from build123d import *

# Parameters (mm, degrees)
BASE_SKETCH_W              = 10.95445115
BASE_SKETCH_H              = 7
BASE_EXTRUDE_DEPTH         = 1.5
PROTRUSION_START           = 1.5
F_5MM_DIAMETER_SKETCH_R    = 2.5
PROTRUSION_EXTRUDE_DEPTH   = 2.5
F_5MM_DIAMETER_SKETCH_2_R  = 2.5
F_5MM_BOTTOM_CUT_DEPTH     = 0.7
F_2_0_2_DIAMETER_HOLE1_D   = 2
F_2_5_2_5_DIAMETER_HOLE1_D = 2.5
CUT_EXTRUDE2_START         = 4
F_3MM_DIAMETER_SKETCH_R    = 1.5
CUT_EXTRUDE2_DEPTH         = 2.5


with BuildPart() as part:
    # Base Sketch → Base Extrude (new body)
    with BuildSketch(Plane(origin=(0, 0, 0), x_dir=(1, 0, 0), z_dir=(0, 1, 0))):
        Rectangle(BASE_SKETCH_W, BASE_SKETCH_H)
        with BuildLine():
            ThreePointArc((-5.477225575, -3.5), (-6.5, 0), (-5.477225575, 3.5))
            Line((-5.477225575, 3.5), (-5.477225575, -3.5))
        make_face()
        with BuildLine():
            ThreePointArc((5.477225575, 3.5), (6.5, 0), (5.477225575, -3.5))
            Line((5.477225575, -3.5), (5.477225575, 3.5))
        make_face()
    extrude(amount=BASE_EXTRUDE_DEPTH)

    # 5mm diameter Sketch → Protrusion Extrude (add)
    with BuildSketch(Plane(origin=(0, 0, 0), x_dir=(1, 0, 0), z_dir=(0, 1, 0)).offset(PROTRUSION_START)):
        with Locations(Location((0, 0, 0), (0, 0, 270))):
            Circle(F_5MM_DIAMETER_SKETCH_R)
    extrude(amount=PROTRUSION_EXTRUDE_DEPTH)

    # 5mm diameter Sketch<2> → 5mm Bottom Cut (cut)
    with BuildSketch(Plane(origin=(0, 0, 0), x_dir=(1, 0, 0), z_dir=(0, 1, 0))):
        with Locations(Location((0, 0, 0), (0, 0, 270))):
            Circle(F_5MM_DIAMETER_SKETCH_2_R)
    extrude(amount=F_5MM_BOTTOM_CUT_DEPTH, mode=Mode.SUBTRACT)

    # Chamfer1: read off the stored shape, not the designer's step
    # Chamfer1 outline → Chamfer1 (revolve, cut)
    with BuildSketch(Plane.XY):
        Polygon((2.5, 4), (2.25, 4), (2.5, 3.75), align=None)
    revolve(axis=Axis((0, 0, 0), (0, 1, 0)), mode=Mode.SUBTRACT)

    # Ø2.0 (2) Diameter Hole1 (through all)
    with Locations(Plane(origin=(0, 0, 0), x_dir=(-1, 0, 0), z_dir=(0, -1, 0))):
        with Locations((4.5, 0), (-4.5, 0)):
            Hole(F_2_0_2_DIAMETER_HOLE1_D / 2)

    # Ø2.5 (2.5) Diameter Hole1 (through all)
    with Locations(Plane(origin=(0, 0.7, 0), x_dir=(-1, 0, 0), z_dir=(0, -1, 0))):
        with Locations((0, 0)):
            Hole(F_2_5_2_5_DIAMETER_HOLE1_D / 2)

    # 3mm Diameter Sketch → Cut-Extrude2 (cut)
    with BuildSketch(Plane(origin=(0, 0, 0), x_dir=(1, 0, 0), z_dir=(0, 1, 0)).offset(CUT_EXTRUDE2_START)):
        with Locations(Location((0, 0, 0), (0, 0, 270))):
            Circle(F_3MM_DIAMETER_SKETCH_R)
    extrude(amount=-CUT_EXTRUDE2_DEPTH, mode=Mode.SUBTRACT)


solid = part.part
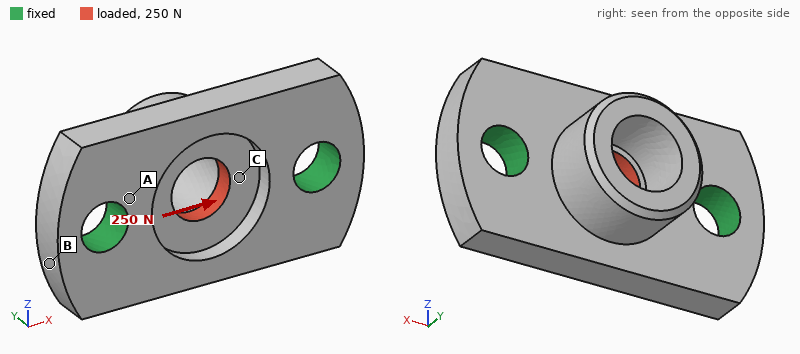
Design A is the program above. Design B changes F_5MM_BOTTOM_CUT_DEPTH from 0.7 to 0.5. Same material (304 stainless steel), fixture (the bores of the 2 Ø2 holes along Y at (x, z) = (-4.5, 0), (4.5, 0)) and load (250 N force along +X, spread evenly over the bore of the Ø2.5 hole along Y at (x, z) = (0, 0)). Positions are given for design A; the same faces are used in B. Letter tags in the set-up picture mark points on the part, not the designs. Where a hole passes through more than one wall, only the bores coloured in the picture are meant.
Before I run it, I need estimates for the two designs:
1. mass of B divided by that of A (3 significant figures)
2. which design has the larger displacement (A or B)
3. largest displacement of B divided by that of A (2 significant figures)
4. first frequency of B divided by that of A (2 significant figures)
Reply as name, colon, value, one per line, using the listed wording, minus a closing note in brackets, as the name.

mass of B divided by that of A: 1.02
which design has the larger displacement: A
largest displacement of B divided by that of A: 0.86
first frequency of B divided by that of A: 1.0
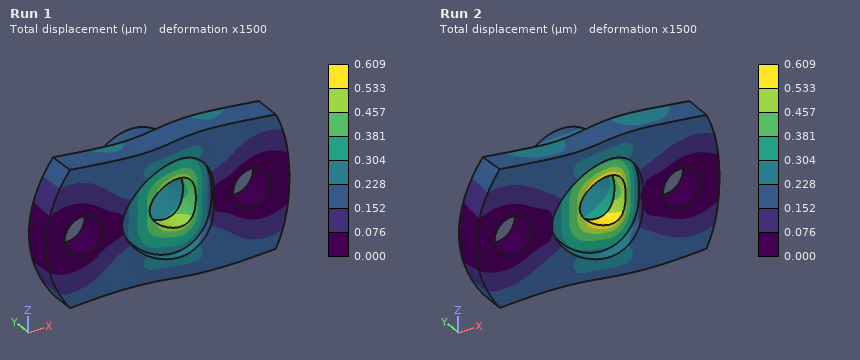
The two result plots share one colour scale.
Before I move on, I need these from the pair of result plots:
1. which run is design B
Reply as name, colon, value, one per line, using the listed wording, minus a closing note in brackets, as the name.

which run is design B: Run 1
